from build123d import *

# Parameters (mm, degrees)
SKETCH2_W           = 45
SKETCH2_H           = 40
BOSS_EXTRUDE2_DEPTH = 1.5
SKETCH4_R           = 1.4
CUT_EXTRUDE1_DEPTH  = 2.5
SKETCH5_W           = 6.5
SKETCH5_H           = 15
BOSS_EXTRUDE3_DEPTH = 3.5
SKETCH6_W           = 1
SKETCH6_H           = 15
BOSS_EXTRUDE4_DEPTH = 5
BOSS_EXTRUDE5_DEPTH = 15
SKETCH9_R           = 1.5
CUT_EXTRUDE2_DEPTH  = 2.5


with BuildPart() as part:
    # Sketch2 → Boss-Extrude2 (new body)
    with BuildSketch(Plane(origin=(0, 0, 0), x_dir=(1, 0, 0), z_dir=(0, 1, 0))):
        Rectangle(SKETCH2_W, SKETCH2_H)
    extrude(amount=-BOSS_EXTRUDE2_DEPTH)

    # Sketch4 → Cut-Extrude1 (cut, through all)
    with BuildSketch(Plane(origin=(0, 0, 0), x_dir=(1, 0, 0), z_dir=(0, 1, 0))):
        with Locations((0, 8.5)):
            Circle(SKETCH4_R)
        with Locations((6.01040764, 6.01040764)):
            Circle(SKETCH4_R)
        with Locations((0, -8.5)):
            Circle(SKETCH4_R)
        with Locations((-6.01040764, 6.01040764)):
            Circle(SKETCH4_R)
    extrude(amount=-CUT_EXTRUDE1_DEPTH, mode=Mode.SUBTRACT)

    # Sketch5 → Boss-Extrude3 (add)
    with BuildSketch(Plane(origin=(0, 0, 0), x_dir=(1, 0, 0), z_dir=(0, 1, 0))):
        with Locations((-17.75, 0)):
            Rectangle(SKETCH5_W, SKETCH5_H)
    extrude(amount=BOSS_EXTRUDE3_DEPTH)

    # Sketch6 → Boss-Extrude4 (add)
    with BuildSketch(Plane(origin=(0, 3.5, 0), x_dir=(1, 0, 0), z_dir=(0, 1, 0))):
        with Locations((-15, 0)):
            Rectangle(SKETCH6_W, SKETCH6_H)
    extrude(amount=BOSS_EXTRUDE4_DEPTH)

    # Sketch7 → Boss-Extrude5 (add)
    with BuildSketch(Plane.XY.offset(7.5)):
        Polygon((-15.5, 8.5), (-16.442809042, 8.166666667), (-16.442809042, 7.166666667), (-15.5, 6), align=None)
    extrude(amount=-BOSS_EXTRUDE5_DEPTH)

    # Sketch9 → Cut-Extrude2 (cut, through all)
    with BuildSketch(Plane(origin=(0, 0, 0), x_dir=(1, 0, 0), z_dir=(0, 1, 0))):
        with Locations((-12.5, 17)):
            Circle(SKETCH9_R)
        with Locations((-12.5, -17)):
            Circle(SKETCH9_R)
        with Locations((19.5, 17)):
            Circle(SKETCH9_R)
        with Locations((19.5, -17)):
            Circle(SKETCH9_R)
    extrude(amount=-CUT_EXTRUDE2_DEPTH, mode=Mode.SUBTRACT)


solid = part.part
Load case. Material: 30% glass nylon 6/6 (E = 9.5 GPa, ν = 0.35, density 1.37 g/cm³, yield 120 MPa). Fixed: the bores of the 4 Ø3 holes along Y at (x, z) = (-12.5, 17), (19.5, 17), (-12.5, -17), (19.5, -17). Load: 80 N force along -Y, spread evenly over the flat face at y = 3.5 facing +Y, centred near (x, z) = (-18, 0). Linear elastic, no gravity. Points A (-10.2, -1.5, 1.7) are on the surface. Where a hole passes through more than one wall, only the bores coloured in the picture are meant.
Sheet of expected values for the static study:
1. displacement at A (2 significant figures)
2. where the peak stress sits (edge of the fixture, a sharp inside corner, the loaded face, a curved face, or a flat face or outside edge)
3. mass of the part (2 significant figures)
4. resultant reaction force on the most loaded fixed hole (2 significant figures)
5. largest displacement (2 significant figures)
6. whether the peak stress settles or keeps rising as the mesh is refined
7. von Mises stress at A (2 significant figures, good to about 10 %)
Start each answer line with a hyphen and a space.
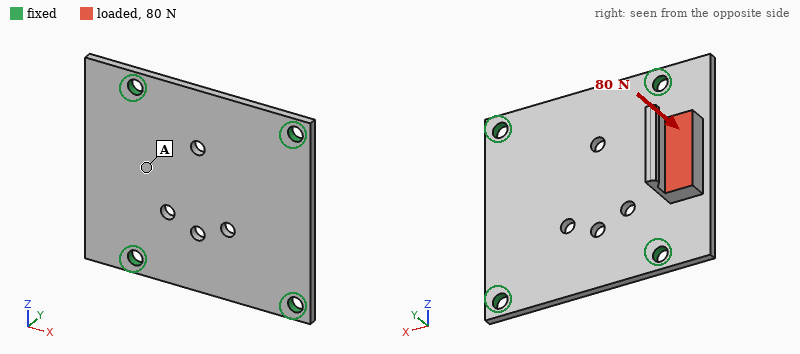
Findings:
- 0.065 mm
- edge of the fixture
- 4.2 g
- 47 N
- 0.31 mm
- keeps rising
- 9.3 MPa
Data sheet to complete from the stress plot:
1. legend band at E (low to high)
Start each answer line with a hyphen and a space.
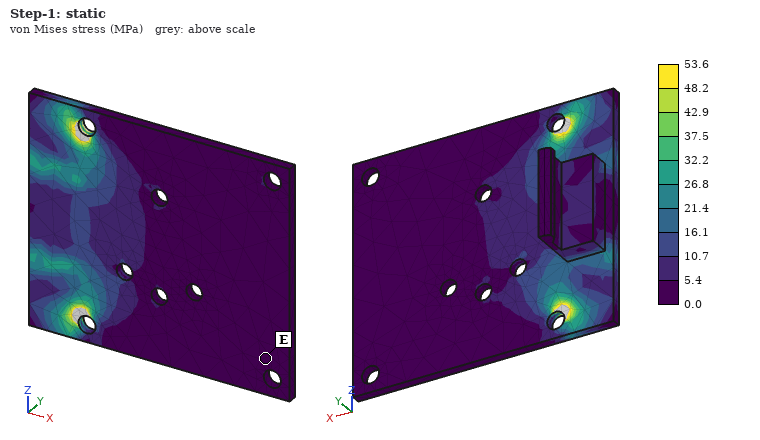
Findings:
- 0.0 to 5.4 MPa
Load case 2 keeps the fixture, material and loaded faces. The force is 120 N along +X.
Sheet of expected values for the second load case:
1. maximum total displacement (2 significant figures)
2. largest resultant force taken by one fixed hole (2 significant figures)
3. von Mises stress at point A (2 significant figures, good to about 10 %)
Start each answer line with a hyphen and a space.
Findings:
- 0.31 mm
- 38 N
- 19 MPa
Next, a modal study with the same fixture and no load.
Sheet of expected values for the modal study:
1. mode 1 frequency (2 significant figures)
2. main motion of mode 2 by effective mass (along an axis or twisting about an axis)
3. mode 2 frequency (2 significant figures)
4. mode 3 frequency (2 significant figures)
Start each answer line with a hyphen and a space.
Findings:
- 2700 Hz
- along Y
- 3000 Hz
- 4500 Hz
